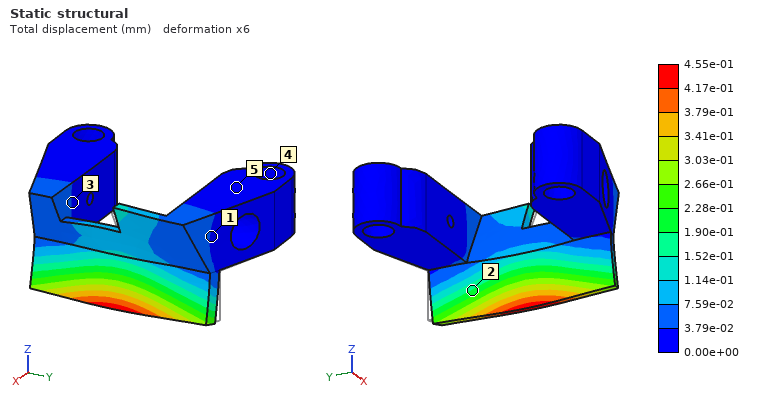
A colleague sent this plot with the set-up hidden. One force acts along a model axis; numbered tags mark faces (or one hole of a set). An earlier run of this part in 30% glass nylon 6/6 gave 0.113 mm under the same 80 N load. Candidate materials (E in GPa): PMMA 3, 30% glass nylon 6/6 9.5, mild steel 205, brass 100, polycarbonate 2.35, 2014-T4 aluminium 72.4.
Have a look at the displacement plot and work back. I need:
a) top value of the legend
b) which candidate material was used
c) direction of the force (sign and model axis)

4.55e-01 mm
polycarbonate
+X
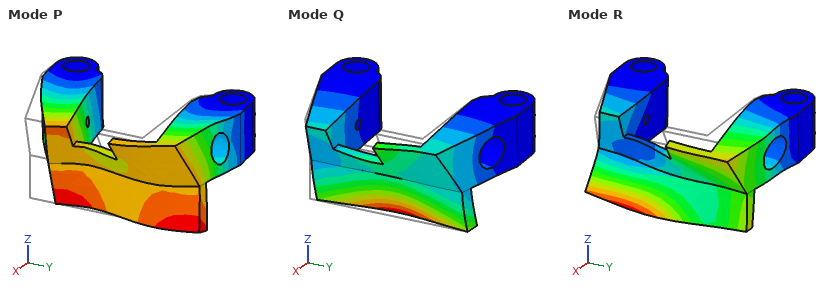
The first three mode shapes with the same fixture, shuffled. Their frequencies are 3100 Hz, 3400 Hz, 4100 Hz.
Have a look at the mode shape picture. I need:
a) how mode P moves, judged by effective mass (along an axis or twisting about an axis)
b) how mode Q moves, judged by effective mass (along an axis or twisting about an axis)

along Y
along Z
